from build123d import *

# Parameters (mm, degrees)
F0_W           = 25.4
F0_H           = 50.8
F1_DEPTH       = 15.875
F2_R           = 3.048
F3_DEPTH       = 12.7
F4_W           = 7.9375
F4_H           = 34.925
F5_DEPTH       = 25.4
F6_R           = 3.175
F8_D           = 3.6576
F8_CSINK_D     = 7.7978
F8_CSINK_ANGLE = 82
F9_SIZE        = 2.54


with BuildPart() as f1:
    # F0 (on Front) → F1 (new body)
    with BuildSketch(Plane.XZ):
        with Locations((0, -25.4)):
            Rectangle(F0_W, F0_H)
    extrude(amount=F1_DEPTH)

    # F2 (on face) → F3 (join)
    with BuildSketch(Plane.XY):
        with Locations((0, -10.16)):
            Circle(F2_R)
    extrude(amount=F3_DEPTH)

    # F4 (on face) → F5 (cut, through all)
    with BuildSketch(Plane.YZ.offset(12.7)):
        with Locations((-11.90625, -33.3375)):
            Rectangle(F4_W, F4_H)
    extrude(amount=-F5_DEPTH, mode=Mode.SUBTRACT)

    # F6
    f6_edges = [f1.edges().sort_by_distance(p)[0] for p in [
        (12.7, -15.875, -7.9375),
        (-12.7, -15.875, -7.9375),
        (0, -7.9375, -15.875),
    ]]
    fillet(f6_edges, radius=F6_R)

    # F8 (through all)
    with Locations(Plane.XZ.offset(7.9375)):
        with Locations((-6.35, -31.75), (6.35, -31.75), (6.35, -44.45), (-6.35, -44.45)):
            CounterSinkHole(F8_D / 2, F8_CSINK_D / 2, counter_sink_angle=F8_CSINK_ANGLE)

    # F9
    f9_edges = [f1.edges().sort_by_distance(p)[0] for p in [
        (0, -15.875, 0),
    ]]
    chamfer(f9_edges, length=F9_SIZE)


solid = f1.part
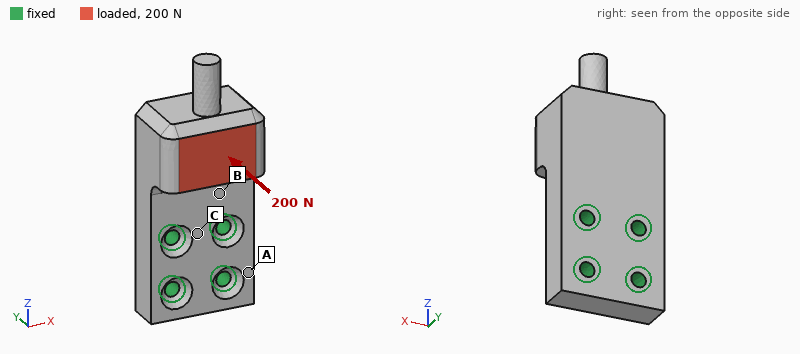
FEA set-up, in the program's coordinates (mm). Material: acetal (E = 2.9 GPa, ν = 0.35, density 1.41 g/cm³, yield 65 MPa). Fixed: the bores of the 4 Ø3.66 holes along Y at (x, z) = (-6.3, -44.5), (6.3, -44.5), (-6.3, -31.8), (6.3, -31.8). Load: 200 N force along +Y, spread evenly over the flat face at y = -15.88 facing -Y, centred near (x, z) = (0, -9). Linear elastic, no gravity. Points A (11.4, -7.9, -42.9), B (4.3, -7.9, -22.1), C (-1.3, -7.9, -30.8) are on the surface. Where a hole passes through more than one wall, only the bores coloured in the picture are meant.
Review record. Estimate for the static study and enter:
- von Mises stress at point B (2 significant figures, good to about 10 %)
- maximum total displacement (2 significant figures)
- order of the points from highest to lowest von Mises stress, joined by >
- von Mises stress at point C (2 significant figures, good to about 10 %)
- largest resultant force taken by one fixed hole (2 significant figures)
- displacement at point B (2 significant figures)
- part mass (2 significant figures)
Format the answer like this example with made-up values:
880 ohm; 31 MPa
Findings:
8.9 MPa; 0.76 mm; C > B > A; 13 MPa; 170 N; 0.12 mm; 19 g
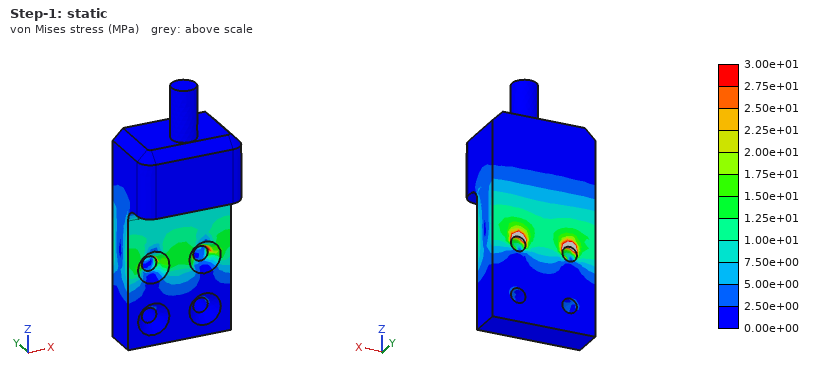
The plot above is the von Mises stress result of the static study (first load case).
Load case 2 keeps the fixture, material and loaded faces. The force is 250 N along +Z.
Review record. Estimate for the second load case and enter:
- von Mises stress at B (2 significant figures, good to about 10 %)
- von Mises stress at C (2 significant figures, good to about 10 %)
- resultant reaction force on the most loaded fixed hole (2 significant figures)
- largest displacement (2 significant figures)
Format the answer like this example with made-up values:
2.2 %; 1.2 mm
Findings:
12 MPa; 10 MPa; 87 N; 0.74 mm
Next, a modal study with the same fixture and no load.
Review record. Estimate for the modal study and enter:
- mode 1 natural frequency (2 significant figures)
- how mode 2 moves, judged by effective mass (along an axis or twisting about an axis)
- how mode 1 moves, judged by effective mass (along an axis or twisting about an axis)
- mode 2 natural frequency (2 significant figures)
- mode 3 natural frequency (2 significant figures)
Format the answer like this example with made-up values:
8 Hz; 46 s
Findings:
1000 Hz; along X; along Y; 2500 Hz; 3400 Hz
